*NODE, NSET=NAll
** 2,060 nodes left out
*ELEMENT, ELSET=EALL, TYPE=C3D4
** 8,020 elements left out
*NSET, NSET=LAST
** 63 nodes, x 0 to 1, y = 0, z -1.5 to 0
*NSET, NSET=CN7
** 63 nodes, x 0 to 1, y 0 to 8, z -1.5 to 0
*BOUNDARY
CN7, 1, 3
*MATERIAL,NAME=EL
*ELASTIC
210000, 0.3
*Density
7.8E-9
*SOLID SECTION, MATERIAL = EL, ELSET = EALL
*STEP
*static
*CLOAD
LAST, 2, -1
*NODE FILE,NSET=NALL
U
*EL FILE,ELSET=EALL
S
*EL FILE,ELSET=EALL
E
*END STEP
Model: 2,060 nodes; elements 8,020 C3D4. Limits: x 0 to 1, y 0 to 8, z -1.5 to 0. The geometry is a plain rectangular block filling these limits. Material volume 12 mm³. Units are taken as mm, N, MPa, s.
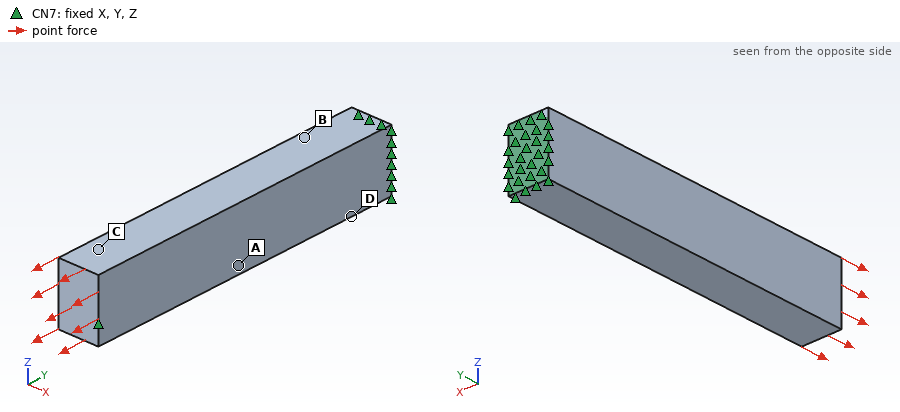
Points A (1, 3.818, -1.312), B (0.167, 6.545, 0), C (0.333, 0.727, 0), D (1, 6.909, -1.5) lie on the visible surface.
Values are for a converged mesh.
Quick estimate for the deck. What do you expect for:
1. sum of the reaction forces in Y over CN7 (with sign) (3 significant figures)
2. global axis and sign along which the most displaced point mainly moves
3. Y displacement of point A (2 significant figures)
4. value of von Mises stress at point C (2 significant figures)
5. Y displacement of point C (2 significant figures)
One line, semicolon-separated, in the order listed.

63.0 N; -Y; -8.2e-04 mm; 46 MPa; -0.0014 mm
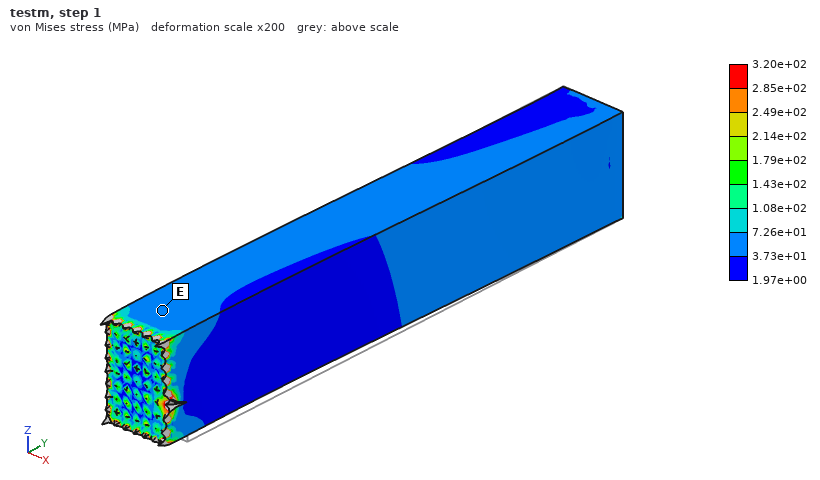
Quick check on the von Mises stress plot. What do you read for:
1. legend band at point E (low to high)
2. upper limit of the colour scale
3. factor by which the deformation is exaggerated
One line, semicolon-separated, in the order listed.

3.73e+01 to 7.26e+01 MPa; 3.20e+02 MPa; 200
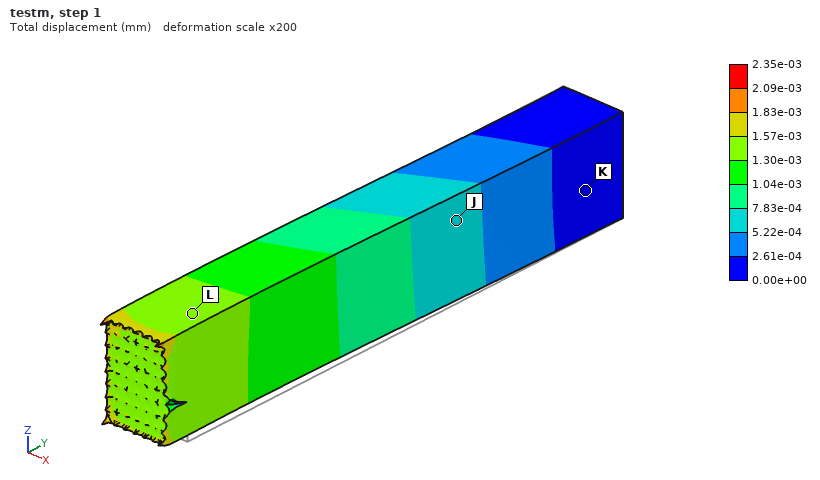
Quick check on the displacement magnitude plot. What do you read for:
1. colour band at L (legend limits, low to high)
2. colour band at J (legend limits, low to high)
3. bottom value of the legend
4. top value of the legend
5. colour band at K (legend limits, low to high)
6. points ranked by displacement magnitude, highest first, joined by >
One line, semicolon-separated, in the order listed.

1.30e-03 to 1.57e-03 mm; 5.22e-04 to 7.83e-04 mm; 0.00e+00 mm; 2.35e-03 mm; 0.00e+00 to 2.61e-04 mm; L > J > K
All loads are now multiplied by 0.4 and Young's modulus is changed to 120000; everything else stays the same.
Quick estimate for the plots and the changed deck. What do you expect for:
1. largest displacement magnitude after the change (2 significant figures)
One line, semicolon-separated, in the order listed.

0.0016 mm
